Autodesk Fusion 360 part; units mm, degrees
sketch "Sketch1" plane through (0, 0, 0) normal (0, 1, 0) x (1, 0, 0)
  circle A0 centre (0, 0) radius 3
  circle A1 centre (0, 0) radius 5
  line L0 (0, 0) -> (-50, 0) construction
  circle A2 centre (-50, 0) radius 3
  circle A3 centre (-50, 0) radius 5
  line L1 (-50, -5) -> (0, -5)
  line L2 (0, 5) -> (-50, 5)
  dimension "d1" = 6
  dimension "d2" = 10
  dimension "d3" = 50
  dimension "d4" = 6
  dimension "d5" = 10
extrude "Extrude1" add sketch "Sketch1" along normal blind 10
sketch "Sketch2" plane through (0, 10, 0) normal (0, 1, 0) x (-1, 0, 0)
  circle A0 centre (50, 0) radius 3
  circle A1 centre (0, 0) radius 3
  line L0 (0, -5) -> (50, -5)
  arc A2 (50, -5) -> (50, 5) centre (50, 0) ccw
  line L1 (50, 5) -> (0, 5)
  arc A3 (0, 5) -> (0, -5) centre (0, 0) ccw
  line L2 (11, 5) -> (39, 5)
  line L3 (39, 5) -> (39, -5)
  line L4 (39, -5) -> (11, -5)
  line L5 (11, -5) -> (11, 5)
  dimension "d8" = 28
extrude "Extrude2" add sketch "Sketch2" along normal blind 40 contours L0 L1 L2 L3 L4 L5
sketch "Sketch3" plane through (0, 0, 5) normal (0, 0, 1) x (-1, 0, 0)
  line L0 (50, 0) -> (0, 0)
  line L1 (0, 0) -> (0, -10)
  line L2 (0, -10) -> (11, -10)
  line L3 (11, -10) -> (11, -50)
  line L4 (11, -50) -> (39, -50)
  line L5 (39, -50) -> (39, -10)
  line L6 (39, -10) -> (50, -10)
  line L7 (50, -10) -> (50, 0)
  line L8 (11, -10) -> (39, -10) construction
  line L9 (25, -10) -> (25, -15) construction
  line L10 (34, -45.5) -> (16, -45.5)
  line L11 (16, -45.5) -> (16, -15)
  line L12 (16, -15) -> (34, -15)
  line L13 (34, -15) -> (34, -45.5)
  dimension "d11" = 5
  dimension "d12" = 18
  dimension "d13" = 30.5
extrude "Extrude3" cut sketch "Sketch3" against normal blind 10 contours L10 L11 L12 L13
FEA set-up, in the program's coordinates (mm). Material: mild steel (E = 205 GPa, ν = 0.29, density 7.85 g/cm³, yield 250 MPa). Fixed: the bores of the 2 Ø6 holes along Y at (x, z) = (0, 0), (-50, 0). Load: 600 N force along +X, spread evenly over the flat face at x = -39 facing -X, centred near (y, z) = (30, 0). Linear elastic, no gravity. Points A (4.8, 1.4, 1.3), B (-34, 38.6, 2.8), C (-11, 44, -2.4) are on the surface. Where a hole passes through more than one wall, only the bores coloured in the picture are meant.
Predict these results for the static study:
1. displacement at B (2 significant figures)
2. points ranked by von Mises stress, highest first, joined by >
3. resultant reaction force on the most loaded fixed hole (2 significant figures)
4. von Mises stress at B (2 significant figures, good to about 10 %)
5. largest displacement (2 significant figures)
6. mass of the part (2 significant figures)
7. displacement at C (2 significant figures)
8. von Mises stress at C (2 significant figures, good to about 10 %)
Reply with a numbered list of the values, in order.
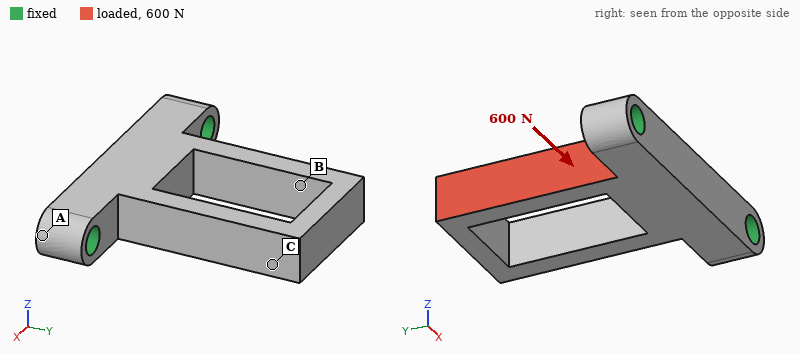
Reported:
1. 31 µm
2. B > C > A
3. 510 N
4. 41 MPa
5. 37 µm
6. 86 g
7. 33 µm
8. 30 MPa
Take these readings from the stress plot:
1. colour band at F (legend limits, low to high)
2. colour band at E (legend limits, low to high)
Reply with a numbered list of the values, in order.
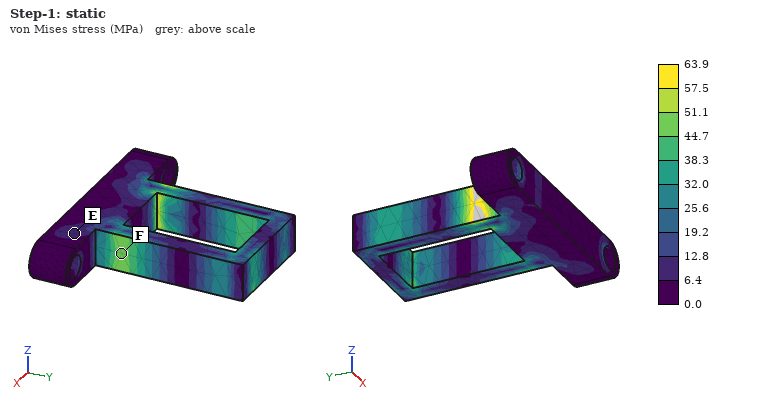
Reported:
1. 44.7 to 51.1 MPa
2. 6.4 to 12.8 MPa
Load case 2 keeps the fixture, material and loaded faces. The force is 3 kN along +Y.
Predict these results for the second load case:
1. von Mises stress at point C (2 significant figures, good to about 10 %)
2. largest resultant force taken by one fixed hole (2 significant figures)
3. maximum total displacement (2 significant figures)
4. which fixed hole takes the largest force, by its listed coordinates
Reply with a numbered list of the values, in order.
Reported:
1. 21 MPa
2. 2.7 kN
3. 41 µm
4. (-50, 0)
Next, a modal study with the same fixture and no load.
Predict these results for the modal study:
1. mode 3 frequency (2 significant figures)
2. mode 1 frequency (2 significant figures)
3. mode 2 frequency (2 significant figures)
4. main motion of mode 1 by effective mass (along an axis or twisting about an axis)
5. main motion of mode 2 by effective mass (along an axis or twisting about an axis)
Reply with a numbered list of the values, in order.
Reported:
1. 6300 Hz
2. 2600 Hz
3. 3400 Hz
4. along Z
5. along X
